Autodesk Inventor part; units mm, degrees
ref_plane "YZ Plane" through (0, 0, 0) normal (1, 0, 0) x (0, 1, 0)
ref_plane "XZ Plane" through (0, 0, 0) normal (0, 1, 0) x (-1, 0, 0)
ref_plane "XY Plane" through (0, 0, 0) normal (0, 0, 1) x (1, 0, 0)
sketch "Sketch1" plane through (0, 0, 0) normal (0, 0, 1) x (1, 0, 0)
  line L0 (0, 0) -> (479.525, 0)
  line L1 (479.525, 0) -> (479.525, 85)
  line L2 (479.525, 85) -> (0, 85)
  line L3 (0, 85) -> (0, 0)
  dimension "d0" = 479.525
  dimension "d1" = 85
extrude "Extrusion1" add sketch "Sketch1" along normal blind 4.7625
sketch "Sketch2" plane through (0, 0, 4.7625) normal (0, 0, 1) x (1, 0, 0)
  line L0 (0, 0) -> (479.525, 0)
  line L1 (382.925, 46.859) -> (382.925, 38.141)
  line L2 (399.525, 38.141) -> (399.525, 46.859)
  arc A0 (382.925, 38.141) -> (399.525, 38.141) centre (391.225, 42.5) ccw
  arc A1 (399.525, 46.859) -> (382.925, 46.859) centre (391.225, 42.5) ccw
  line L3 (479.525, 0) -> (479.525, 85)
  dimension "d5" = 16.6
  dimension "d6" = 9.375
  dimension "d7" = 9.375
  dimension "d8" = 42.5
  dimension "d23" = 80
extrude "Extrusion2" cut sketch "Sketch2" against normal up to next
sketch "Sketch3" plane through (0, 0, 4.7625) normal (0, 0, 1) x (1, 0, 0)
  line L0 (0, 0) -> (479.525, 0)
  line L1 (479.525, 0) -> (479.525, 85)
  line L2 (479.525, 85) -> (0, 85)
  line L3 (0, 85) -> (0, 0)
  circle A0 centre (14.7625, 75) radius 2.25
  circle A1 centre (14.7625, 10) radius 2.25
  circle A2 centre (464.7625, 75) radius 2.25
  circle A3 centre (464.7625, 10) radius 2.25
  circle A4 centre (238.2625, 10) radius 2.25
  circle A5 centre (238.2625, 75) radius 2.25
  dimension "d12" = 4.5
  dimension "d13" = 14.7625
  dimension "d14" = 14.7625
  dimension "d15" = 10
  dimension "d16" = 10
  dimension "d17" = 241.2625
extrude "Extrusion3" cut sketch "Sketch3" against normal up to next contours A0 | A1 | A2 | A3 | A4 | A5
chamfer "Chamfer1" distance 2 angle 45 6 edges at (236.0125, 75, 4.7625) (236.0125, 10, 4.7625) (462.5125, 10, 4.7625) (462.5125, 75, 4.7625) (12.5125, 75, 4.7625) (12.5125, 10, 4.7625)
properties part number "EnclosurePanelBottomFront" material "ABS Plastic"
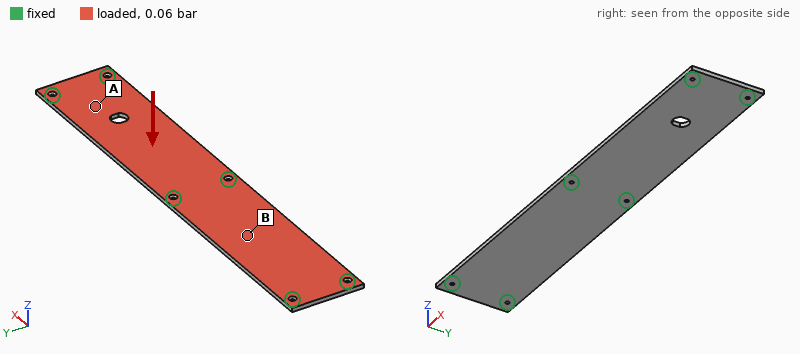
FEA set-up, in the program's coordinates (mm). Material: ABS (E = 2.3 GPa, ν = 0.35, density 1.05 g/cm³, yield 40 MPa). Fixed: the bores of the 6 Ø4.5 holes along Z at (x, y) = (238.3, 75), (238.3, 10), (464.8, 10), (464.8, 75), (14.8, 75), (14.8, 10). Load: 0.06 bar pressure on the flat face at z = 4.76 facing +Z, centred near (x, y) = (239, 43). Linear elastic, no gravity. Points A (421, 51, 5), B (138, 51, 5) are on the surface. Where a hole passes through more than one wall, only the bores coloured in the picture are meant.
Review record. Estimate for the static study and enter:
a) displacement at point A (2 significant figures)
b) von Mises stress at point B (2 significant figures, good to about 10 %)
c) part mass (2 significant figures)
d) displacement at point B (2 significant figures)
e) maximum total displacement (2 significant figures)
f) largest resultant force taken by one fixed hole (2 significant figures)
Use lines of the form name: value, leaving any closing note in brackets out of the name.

displacement at point A: 1.1 mm
von Mises stress at point B: 3.2 MPa
part mass: 200 g
displacement at point B: 2.0 mm
maximum total displacement: 2.3 mm
largest resultant force taken by one fixed hole: 71 N
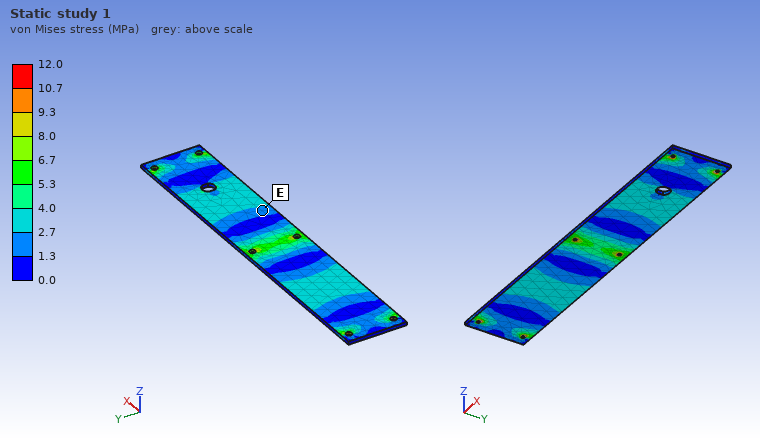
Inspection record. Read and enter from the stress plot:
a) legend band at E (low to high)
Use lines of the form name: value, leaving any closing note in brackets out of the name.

legend band at E: 1.3 to 2.7 MPa
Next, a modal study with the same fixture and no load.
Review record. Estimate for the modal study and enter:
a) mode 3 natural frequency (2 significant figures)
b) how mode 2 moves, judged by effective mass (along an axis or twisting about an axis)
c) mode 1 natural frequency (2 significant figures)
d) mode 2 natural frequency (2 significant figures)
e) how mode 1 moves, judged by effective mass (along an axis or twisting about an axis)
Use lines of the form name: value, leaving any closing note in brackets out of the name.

mode 3 natural frequency: 270 Hz
how mode 2 moves, judged by effective mass: along Z
mode 1 natural frequency: 120 Hz
mode 2 natural frequency: 130 Hz
how mode 1 moves, judged by effective mass: twisting about Y
